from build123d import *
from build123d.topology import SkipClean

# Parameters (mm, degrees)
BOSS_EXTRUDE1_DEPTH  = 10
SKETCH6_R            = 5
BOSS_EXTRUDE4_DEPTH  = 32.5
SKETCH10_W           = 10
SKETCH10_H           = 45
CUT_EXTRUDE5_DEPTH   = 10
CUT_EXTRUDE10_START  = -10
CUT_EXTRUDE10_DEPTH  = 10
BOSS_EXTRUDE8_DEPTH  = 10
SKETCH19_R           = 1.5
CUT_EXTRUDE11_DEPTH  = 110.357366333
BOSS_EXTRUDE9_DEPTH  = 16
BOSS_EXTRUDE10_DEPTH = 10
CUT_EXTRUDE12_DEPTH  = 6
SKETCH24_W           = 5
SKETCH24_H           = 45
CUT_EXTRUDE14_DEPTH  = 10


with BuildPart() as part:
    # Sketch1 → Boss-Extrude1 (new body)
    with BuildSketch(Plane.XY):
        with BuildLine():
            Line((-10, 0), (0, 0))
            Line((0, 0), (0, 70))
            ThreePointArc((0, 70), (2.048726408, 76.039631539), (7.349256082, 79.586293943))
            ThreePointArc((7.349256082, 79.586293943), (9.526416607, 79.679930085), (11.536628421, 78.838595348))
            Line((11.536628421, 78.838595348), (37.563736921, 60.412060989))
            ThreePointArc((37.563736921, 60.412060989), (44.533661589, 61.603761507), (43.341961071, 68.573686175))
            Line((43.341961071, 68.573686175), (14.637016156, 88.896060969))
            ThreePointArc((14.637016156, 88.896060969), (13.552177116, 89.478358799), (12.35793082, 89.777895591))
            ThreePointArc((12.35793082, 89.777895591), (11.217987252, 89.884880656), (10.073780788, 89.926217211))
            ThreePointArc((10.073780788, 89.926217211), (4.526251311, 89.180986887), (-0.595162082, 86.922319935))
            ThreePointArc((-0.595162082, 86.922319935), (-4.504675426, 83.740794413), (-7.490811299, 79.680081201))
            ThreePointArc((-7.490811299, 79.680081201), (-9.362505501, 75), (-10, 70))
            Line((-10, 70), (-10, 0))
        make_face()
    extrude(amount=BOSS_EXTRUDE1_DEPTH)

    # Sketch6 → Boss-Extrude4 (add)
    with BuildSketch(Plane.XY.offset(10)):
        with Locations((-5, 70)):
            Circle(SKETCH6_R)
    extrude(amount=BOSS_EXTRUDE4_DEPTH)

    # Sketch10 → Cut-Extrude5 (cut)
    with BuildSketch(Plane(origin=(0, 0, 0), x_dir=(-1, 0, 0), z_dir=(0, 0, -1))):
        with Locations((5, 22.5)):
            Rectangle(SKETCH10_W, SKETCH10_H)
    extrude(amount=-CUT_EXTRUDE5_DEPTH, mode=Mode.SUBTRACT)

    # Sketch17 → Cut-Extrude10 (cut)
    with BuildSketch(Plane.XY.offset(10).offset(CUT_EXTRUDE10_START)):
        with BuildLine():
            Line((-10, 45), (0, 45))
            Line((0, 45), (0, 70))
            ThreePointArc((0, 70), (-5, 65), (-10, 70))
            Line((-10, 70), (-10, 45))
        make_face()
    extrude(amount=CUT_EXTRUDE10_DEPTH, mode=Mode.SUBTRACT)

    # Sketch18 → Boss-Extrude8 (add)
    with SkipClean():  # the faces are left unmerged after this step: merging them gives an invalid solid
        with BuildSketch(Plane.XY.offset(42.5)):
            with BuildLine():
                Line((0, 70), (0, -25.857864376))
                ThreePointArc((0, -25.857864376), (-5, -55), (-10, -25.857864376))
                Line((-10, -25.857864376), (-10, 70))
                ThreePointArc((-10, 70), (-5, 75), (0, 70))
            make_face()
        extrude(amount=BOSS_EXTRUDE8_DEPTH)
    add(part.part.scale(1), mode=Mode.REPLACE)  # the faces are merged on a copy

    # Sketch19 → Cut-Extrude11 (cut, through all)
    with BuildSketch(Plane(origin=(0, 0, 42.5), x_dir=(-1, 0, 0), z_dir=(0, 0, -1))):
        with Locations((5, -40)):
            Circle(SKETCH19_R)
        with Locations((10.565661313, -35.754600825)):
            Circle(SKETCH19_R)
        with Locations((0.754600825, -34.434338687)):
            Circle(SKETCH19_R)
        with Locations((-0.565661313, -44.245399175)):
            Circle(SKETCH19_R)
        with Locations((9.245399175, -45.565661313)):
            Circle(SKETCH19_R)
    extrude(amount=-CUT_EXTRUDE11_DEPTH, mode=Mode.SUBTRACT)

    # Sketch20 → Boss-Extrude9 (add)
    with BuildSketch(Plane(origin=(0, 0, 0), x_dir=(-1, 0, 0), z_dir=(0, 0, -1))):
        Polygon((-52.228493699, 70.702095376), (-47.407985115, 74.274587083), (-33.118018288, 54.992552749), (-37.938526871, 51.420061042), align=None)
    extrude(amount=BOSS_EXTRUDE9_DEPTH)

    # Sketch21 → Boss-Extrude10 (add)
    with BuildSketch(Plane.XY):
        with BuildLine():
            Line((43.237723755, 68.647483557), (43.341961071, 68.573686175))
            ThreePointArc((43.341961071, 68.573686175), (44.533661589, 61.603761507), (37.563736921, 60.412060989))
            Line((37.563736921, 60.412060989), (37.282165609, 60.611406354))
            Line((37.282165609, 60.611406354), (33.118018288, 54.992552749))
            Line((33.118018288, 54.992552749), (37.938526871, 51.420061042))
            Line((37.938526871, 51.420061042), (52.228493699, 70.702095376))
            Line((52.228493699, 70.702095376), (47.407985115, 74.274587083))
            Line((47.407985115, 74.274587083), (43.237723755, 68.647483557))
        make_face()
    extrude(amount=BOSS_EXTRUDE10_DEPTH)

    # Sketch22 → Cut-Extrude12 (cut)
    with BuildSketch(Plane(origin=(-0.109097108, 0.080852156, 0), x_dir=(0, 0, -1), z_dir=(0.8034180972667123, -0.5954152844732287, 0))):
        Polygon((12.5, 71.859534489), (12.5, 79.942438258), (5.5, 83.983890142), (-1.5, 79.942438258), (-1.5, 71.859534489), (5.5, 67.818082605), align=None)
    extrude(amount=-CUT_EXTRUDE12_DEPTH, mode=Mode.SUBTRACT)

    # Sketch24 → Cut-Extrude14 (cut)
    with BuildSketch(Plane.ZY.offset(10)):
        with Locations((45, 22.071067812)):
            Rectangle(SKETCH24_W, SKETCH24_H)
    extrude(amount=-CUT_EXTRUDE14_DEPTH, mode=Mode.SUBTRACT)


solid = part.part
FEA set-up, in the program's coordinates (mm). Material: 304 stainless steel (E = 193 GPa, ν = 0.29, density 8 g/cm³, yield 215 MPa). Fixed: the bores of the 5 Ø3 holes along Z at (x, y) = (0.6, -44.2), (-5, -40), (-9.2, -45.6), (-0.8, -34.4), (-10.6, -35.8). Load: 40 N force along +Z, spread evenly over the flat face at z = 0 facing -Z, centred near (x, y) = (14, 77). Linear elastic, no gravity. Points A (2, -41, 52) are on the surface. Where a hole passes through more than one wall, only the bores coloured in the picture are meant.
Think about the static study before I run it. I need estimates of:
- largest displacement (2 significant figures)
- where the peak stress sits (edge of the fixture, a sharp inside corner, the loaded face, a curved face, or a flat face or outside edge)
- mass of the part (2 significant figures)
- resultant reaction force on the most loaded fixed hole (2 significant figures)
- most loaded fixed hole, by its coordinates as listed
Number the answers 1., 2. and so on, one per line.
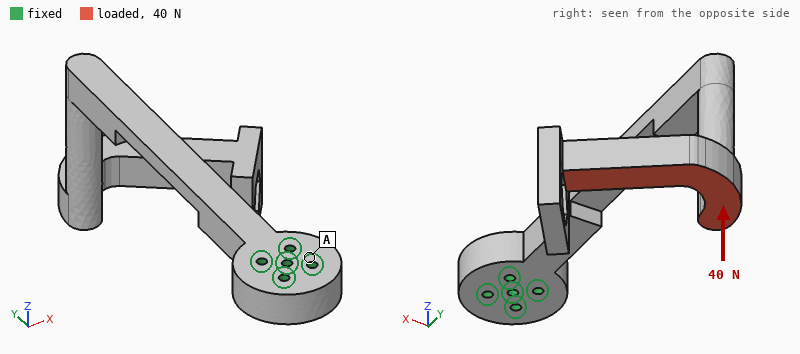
1. 0.65 mm
2. a flat face or outside edge
3. 210 g
4. 130 N
5. (-0.8, -34.4)
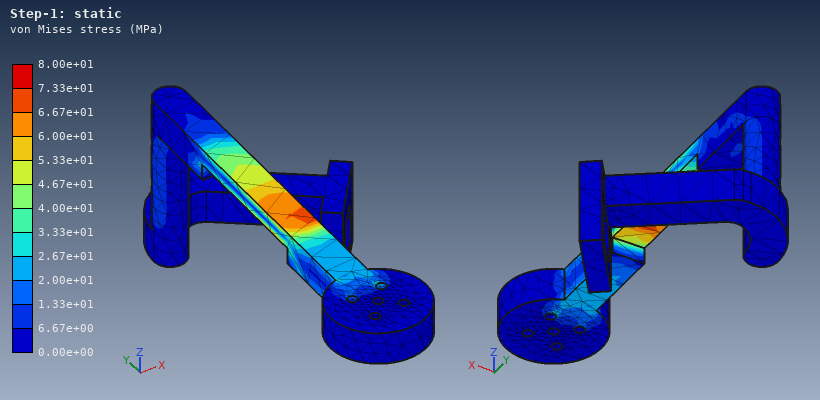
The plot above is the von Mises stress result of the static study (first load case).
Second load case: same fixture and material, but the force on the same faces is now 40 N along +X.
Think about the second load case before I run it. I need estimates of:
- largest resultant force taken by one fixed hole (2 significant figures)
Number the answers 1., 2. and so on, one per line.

1. 320 N
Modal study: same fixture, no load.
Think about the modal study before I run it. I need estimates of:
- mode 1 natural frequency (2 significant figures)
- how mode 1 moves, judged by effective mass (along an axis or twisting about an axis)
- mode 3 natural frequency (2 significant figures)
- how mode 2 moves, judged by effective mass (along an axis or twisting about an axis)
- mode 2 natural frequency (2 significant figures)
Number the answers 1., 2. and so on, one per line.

1. 130 Hz
2. along Z
3. 460 Hz
4. along X
5. 170 Hz
